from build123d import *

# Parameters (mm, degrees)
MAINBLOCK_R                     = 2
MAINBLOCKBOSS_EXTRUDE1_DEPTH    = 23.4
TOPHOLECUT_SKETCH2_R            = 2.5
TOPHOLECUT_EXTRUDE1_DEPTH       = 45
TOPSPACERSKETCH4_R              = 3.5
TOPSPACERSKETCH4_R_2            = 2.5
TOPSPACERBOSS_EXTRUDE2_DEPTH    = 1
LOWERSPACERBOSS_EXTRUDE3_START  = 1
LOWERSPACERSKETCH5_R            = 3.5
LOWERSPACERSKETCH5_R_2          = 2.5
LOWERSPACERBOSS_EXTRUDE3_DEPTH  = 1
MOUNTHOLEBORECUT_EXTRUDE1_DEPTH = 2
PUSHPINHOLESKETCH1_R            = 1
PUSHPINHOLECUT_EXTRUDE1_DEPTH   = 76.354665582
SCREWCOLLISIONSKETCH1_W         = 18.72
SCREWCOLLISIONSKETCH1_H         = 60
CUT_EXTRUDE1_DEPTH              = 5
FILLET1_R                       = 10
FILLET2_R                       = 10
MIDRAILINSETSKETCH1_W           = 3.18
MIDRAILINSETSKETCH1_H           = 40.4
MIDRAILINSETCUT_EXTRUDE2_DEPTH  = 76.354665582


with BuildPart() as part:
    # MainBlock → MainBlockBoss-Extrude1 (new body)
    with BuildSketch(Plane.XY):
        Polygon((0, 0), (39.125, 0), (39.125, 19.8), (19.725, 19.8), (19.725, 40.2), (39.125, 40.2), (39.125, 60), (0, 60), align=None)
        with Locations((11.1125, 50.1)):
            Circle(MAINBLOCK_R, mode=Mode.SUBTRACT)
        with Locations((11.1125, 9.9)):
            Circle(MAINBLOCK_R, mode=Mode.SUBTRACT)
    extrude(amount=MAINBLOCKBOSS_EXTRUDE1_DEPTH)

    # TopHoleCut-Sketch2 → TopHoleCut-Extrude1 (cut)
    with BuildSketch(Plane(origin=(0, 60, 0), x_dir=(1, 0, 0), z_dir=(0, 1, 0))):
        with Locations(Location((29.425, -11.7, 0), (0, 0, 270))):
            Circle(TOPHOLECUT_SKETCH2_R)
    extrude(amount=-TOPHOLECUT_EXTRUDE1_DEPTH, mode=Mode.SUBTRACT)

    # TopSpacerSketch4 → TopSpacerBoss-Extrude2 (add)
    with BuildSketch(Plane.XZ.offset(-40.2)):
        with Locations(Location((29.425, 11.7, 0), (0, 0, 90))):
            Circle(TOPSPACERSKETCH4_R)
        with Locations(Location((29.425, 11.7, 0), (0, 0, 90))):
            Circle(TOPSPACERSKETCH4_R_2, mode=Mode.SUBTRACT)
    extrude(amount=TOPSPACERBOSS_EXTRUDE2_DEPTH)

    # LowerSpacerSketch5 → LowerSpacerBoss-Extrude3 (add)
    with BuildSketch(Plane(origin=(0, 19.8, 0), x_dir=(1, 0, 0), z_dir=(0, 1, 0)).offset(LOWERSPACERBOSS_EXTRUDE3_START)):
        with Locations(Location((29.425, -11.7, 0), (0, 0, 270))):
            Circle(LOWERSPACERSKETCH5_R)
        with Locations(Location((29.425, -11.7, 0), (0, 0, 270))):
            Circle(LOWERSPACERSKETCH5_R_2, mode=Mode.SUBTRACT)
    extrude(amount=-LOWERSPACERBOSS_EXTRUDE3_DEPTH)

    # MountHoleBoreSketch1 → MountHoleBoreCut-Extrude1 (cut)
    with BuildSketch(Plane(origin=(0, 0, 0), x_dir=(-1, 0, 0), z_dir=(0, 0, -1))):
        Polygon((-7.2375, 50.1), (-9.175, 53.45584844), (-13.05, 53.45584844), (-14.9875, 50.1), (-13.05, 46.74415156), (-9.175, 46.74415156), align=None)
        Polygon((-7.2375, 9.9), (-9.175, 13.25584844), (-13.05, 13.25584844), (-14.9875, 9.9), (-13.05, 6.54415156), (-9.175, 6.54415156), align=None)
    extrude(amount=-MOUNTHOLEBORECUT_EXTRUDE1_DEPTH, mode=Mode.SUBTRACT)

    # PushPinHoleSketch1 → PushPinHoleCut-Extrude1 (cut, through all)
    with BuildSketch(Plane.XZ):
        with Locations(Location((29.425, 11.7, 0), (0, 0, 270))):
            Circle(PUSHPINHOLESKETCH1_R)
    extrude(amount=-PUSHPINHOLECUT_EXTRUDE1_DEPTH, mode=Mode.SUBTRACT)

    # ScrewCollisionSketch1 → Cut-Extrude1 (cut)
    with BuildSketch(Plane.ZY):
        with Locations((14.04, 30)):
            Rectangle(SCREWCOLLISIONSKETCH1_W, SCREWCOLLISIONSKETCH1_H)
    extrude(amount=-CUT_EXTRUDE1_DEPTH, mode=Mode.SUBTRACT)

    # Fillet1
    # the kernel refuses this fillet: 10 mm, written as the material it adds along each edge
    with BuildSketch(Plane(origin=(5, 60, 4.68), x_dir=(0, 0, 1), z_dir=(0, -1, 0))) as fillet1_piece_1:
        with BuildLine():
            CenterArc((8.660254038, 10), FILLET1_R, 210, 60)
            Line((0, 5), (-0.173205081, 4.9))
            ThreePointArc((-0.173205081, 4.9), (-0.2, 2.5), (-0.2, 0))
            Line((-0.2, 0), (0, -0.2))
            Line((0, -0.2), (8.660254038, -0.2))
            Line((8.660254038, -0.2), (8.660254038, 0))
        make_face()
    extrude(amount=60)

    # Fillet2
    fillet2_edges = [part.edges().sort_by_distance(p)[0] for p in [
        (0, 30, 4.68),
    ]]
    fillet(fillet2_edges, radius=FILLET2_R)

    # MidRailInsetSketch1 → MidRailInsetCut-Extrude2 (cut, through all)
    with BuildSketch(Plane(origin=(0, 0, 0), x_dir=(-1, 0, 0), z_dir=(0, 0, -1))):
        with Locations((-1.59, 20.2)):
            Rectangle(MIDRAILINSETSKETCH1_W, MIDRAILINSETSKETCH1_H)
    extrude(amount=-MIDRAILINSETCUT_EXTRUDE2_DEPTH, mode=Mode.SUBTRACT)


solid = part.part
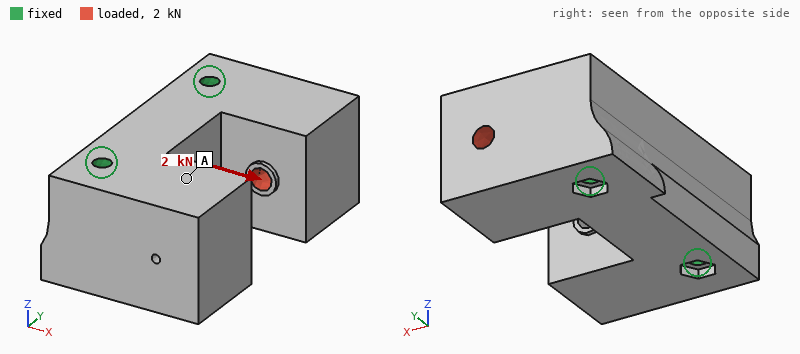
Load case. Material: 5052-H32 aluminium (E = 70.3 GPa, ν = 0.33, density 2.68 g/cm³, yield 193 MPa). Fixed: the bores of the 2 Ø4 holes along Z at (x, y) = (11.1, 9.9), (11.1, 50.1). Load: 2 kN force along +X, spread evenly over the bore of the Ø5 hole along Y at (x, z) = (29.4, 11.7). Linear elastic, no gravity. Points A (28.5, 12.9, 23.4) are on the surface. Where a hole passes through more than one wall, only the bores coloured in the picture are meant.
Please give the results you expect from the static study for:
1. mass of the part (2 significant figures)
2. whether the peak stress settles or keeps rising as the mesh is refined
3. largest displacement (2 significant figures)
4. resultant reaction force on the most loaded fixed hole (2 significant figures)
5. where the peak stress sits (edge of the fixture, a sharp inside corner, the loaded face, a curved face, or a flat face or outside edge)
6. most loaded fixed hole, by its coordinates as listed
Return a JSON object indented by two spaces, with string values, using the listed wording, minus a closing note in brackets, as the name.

{
  "mass of the part": "100 g",
  "whether the peak stress settles or keeps rising as the mesh is refined": "keeps rising",
  "largest displacement": "2.6 µm",
  "resultant reaction force on the most loaded fixed hole": "2.0 kN",
  "where the peak stress sits": "edge of the fixture",
  "most loaded fixed hole, by its coordinates as listed": "(11.1, 50.1)"
}
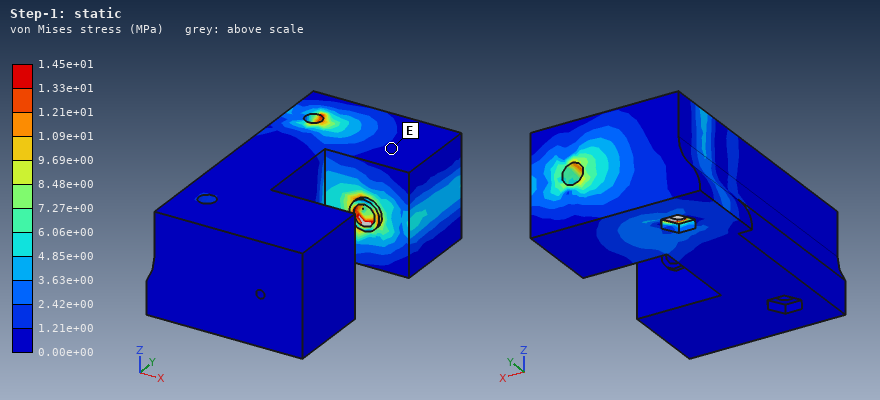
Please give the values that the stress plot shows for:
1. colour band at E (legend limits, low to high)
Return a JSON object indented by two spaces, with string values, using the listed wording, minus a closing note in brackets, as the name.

{
  "colour band at E": "0.00e+00 to 1.21e+00 MPa"
}
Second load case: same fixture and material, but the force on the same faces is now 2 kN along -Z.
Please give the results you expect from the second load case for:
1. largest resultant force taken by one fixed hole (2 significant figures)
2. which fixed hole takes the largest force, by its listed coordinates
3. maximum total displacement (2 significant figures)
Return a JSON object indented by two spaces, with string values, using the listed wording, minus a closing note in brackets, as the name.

{
  "largest resultant force taken by one fixed hole": "1.9 kN",
  "which fixed hole takes the largest force, by its listed coordinates": "(11.1, 50.1)",
  "maximum total displacement": "13 µm"
}
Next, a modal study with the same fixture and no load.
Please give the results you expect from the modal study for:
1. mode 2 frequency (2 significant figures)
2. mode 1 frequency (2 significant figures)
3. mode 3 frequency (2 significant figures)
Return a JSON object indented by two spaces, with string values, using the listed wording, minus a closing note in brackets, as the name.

{
  "mode 2 frequency": "14 kHz",
  "mode 1 frequency": "11 kHz",
  "mode 3 frequency": "14 kHz"
}
